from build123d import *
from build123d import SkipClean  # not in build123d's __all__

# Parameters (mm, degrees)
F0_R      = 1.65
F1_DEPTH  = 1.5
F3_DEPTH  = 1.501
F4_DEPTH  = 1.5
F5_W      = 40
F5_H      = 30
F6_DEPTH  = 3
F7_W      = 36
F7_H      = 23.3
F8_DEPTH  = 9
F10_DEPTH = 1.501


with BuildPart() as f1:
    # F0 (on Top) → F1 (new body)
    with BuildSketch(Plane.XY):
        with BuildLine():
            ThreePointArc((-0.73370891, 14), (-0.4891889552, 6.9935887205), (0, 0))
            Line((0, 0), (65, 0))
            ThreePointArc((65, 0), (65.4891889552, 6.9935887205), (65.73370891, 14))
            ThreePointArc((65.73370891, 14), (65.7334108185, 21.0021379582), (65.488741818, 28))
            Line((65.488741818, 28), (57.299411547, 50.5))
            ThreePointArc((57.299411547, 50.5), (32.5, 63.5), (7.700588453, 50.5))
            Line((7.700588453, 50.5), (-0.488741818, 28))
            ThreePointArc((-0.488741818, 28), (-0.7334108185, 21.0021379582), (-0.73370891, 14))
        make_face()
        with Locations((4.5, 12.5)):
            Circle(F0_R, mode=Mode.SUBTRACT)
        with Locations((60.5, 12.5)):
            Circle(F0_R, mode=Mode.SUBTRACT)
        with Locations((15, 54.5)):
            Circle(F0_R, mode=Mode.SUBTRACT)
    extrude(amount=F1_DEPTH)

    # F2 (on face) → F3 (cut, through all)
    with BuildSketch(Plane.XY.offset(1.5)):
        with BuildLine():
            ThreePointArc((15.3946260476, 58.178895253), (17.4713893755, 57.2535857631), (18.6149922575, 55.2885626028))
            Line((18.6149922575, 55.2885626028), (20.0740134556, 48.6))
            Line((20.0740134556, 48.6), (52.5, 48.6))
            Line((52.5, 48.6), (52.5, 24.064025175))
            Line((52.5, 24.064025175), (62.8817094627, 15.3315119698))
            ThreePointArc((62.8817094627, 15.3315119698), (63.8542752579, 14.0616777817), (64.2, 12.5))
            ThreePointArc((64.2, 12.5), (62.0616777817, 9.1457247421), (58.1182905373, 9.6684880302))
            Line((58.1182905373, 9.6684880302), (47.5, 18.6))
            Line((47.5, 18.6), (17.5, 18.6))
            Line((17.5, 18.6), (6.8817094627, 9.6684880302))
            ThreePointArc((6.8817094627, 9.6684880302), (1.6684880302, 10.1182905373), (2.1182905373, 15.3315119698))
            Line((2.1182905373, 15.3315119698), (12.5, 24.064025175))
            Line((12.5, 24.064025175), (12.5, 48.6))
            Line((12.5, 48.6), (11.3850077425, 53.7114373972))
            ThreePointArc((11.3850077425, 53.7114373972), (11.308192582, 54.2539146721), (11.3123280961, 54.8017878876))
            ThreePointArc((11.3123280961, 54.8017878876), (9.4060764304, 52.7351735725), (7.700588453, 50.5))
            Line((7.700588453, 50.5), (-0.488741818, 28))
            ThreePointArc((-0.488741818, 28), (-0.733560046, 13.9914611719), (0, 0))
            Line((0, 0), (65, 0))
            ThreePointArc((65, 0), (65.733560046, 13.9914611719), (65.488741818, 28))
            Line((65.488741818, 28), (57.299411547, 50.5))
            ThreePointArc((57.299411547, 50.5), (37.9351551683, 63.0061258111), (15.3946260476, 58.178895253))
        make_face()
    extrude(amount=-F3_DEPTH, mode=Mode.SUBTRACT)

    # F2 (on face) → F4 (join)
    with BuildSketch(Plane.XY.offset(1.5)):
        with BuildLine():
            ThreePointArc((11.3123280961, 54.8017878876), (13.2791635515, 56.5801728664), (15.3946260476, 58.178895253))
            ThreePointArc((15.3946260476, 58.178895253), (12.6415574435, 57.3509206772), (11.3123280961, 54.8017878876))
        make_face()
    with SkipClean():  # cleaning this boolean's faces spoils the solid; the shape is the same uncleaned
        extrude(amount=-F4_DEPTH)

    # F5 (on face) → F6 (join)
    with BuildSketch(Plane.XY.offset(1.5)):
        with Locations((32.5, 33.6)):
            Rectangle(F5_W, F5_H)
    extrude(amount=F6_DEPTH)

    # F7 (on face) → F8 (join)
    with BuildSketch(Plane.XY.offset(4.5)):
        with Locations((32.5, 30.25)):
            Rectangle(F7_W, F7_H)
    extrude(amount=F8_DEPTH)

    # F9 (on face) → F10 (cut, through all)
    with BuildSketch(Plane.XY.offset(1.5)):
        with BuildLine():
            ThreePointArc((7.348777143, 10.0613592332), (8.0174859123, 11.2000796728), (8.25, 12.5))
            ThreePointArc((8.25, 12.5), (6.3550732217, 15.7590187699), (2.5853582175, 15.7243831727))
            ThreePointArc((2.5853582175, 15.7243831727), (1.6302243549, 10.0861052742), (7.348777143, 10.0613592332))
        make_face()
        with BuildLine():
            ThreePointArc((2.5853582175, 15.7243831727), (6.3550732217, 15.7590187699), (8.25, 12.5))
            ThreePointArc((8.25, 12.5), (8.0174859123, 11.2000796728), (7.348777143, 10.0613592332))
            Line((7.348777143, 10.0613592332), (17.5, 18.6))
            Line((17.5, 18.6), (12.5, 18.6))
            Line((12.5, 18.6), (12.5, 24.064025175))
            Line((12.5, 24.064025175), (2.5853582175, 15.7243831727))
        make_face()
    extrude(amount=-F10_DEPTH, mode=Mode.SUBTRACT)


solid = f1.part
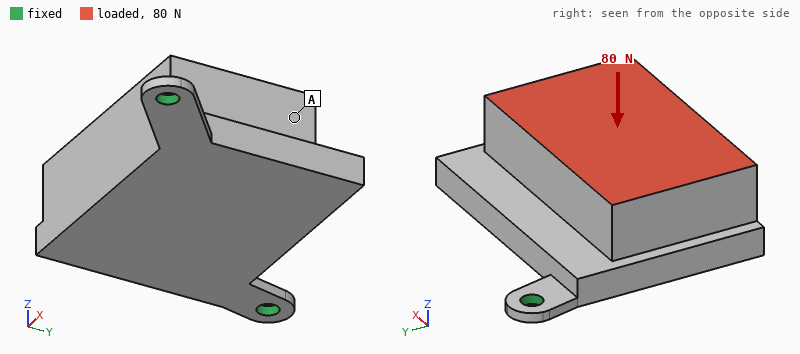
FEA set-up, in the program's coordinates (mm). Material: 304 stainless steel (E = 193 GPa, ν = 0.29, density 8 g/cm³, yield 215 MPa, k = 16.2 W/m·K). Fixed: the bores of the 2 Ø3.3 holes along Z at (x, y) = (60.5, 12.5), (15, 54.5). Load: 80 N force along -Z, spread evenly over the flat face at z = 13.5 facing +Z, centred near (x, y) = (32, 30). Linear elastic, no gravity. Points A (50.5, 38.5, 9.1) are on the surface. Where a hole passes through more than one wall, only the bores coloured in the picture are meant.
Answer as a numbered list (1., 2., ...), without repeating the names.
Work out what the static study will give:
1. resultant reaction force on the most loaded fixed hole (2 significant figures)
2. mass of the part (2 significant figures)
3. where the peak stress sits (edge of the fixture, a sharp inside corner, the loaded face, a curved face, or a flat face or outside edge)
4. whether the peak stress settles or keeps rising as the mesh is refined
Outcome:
1. 48 N
2. 110 g
3. edge of the fixture
4. keeps rising
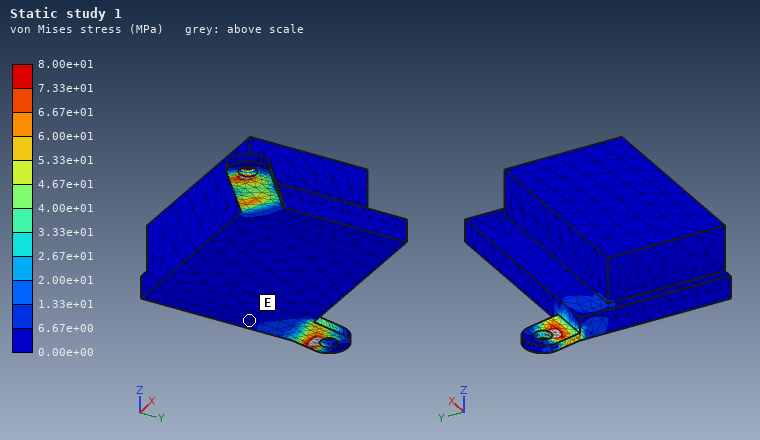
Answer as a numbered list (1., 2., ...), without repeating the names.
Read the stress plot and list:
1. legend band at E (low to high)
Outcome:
1. 0.00e+00 to 6.67e+00 MPa
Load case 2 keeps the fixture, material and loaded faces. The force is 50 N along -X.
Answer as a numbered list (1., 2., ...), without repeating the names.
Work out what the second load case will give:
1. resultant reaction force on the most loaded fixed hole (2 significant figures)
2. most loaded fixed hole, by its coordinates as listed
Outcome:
1. 35 N
2. (60.5, 12.5)
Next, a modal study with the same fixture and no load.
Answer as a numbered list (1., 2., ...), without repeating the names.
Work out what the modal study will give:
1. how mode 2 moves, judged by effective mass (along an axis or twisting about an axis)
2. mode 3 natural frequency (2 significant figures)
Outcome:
1. along Z
2. 4200 Hz
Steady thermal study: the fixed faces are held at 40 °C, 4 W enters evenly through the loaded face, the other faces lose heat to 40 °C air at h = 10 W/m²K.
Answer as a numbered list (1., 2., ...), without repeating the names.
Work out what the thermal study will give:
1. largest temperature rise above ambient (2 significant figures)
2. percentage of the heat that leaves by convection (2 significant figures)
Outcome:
1. 63 K
2. 49 %
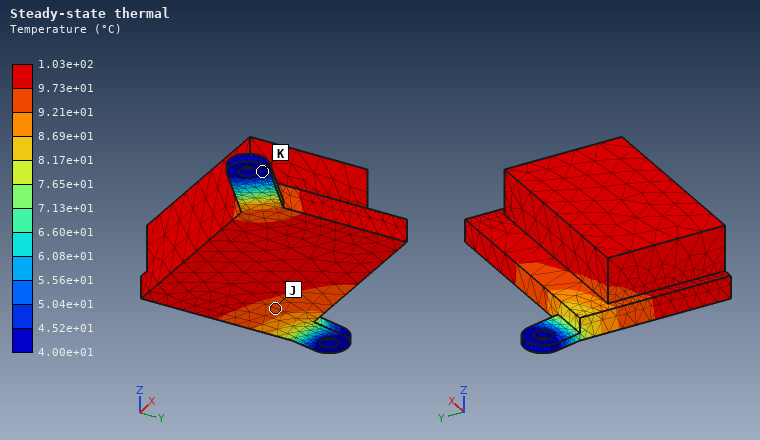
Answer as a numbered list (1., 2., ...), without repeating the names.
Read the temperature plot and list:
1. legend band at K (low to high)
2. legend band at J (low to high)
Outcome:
1. 4.00e+01 to 4.52e+01 °C
2. 9.21e+01 to 9.73e+01 °C
